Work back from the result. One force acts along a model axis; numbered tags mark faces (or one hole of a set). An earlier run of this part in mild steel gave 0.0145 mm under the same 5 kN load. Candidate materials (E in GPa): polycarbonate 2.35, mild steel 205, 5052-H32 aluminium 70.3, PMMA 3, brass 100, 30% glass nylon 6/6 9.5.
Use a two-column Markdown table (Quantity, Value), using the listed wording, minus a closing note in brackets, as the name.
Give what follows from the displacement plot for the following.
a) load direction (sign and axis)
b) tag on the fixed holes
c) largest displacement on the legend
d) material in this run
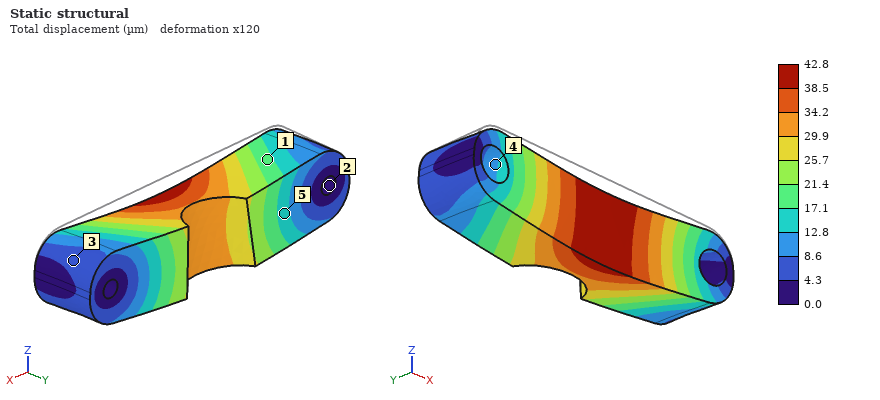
| Quantity | Value |
|---|---|
| load direction | -Z |
| tag on the fixed holes | 2 |
| largest displacement on the legend | 42.8 µm |
| material in this run | 5052-H32 aluminium |
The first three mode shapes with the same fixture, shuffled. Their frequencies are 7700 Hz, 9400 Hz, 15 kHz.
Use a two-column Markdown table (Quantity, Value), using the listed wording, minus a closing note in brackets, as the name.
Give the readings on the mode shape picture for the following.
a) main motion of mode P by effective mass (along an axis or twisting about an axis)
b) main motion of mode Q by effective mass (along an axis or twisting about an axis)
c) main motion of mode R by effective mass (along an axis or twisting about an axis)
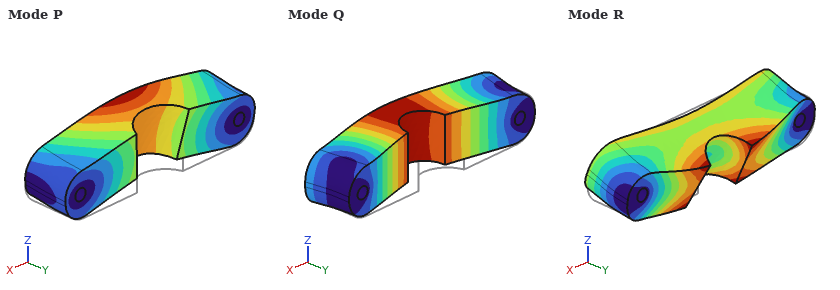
| Quantity | Value |
|---|---|
| main motion of mode P by effective mass | along Z |
| main motion of mode Q by effective mass | along Y |
| main motion of mode R by effective mass | twisting about X |
